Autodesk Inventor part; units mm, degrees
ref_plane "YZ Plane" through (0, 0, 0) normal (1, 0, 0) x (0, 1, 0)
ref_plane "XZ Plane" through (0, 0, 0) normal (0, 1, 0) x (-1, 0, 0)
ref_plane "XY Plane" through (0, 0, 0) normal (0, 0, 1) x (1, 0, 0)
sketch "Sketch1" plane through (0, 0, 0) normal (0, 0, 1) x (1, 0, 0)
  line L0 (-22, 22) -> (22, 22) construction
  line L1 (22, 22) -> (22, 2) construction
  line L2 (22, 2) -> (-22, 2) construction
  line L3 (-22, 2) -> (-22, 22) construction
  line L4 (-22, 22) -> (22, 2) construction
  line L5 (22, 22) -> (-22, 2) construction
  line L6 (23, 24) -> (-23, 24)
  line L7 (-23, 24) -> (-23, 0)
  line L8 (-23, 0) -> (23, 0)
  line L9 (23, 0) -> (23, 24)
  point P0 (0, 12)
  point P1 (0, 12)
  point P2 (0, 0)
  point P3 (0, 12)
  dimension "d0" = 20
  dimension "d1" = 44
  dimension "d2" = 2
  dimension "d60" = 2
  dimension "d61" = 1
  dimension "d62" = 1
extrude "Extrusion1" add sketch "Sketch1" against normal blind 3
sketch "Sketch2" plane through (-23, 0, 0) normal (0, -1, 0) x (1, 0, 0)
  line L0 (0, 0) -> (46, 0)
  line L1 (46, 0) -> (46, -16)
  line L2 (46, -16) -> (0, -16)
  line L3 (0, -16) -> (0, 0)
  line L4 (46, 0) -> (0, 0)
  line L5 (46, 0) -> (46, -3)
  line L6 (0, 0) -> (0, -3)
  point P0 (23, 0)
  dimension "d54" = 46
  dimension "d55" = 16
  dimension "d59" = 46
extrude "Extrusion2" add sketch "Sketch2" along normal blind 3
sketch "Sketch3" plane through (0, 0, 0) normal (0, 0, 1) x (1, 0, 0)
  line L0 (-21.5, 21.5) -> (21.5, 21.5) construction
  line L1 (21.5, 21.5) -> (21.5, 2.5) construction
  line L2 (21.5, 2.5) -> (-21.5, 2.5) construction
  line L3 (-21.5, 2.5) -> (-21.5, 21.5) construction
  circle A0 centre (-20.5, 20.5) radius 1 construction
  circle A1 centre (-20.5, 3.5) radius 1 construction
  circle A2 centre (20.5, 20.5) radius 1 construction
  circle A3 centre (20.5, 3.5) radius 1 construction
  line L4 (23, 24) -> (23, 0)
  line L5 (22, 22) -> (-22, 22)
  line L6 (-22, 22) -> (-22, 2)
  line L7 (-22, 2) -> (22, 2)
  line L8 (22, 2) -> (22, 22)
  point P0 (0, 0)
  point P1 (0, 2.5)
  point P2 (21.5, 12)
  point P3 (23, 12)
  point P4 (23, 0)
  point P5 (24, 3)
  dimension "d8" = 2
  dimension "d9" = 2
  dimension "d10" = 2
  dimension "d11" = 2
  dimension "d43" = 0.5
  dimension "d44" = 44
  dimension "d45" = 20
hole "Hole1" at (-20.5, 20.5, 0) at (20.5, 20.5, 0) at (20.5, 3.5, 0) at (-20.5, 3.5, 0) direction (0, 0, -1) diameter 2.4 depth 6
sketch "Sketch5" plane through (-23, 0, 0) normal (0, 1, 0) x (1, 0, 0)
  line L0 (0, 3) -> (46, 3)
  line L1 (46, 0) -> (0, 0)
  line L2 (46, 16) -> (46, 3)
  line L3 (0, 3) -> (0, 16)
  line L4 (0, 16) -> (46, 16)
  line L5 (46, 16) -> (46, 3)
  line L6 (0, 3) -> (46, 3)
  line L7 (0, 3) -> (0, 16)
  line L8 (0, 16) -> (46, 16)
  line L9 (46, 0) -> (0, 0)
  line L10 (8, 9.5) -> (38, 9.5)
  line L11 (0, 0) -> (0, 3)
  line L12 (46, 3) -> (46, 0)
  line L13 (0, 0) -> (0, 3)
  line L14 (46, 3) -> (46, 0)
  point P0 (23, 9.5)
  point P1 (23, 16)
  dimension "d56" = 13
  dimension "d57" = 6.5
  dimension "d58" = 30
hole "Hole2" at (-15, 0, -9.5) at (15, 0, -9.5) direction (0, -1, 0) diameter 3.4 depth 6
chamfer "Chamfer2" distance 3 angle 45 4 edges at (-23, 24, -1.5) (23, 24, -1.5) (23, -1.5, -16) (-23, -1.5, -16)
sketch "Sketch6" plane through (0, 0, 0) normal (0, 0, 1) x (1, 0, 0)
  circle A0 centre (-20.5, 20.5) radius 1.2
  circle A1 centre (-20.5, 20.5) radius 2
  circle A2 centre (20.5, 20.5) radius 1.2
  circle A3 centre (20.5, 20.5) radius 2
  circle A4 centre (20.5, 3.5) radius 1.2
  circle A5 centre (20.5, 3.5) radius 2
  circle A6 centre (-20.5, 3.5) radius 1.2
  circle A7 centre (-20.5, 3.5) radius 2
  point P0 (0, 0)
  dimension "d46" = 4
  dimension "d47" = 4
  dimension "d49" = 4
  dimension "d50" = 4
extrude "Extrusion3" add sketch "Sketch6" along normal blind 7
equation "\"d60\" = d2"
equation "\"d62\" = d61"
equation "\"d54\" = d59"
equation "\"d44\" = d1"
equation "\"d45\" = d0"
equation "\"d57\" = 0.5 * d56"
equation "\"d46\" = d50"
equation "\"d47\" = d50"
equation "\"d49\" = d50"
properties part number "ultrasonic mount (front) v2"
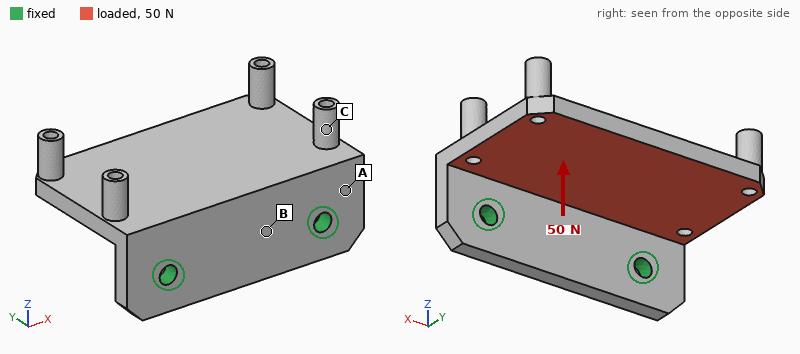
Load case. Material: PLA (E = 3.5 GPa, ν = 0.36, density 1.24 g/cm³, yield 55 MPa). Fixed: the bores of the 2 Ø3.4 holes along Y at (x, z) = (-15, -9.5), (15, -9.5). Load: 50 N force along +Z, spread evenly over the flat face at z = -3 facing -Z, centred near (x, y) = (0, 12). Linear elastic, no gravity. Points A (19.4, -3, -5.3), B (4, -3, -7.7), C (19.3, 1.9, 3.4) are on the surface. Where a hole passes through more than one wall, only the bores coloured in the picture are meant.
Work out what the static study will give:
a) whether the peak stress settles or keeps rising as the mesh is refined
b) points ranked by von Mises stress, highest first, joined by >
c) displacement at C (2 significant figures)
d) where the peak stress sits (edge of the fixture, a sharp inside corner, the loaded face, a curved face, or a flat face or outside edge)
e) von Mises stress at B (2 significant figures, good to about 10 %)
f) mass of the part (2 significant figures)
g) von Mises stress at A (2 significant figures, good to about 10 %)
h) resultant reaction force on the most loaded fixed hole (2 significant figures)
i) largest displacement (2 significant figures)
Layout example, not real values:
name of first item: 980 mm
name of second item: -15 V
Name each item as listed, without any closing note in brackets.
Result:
whether the peak stress settles or keeps rising as the mesh is refined: keeps rising
points ranked by von Mises stress, highest first, joined by >: A > B > C
displacement at C: 0.18 mm
where the peak stress sits: edge of the fixture
von Mises stress at B: 4.7 MPa
mass of the part: 6.9 g
von Mises stress at A: 8.6 MPa
resultant reaction force on the most loaded fixed hole: 26 N
largest displacement: 0.66 mm
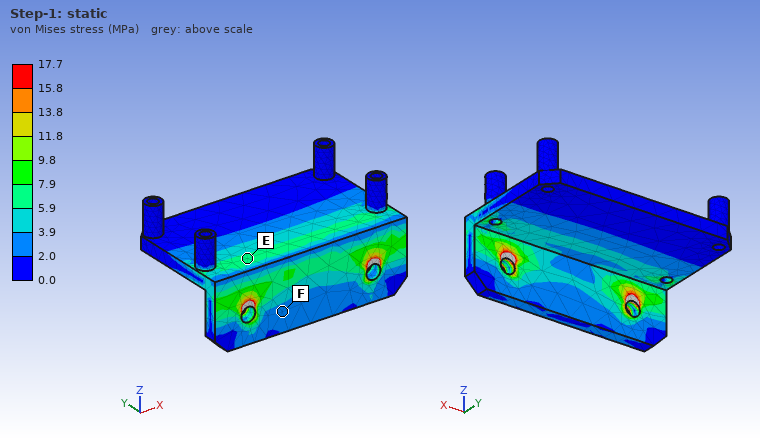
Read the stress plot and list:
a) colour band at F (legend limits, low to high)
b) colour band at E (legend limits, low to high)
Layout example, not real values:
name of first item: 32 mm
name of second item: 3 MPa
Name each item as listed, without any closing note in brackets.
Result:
colour band at F: 2.0 to 3.9 MPa
colour band at E: 5.9 to 7.9 MPa
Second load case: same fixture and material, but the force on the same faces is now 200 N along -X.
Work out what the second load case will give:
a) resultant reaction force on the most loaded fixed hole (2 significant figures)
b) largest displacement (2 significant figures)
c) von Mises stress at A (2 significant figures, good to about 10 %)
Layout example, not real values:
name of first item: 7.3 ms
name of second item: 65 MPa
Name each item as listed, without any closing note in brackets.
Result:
resultant reaction force on the most loaded fixed hole: 140 N
largest displacement: 0.34 mm
von Mises stress at A: 6.7 MPa
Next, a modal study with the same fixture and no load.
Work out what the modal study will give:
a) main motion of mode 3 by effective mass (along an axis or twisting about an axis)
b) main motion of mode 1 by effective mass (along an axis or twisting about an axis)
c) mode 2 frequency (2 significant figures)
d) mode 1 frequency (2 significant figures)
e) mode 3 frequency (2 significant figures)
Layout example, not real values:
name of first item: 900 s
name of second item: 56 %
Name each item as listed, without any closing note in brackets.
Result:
main motion of mode 3 by effective mass: along X
main motion of mode 1 by effective mass: along Z
mode 2 frequency: 1500 Hz
mode 1 frequency: 820 Hz
mode 3 frequency: 2900 Hz
